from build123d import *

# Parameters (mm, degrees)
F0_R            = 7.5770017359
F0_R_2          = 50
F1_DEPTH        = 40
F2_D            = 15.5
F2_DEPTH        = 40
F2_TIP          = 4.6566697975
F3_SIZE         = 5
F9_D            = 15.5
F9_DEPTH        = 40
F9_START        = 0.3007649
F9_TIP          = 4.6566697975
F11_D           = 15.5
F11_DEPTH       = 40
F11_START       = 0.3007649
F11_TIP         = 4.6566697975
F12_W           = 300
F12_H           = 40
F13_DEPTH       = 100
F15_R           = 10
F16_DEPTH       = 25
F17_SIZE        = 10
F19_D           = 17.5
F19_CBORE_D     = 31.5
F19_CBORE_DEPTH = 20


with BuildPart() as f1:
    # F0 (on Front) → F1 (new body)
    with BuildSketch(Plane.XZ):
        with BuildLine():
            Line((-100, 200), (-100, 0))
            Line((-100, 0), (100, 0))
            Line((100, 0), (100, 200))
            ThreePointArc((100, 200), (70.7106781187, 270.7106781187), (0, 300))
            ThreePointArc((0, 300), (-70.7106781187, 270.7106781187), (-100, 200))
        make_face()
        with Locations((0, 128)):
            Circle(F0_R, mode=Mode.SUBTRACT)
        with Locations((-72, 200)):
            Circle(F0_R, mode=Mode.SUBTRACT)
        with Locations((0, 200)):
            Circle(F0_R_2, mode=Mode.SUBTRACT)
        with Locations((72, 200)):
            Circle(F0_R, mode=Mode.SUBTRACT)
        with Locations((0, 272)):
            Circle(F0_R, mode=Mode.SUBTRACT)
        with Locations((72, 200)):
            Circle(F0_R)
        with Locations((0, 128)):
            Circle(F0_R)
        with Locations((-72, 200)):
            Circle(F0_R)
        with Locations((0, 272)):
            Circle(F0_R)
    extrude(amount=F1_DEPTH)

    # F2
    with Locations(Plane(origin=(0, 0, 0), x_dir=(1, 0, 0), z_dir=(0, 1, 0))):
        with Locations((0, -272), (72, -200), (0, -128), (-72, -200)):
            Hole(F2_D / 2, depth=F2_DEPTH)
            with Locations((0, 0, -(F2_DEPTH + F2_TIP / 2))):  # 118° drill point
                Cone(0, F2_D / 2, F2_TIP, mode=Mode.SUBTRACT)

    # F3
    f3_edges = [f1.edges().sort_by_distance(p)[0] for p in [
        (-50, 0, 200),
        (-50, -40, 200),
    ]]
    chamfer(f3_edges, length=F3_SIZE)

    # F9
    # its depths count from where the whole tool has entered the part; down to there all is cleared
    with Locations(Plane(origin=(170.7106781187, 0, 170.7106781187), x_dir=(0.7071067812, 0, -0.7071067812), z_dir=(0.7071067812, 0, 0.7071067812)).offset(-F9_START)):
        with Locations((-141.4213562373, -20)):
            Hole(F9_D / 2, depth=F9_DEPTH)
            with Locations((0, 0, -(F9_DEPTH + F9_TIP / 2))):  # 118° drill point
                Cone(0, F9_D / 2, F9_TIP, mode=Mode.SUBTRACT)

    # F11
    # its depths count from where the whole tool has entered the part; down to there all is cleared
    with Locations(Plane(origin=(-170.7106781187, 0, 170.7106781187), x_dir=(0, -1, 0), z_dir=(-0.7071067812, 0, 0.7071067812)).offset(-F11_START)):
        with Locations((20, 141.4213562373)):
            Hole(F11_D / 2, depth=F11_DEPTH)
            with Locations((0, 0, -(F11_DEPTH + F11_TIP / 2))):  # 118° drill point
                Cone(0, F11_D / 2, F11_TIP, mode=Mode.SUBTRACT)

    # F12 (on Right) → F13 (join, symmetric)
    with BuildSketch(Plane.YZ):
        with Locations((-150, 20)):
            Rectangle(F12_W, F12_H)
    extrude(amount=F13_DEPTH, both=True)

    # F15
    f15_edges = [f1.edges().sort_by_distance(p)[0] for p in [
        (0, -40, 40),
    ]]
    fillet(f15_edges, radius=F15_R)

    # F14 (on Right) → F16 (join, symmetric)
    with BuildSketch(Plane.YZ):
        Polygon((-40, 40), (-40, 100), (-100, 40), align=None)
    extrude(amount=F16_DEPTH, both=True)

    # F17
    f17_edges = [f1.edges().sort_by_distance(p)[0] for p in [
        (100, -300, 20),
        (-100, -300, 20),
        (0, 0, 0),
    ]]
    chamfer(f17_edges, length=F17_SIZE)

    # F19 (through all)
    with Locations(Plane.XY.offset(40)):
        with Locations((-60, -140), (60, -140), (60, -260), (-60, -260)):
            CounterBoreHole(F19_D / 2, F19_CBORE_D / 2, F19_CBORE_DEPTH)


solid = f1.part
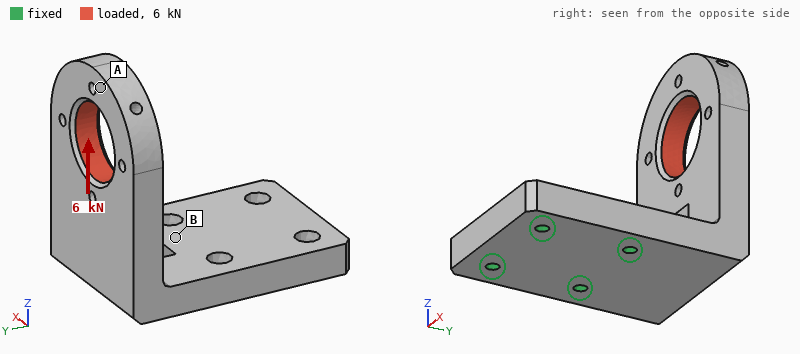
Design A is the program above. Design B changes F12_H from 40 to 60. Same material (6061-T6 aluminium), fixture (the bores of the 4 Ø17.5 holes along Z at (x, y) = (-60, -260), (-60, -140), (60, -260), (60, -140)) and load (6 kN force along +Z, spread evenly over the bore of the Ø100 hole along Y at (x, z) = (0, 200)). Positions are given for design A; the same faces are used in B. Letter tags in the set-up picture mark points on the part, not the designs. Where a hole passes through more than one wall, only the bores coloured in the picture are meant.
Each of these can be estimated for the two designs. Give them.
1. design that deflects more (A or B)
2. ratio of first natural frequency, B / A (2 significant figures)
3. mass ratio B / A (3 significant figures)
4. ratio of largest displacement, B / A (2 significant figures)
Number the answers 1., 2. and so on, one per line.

1. A
2. 1.4
3. 1.27
4. 0.37
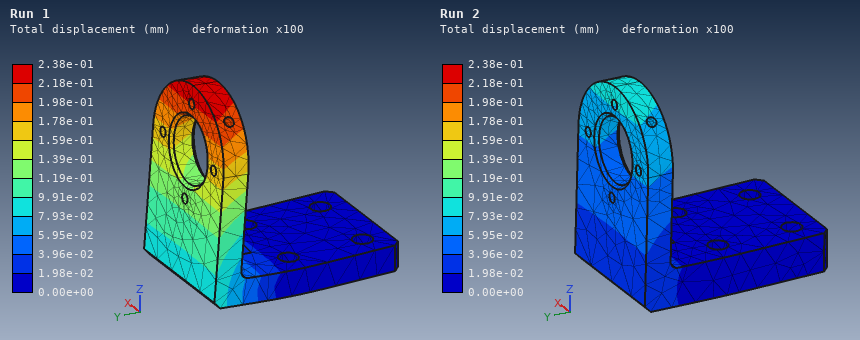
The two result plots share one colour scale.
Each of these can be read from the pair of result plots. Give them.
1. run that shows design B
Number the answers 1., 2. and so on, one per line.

1. Run 2
